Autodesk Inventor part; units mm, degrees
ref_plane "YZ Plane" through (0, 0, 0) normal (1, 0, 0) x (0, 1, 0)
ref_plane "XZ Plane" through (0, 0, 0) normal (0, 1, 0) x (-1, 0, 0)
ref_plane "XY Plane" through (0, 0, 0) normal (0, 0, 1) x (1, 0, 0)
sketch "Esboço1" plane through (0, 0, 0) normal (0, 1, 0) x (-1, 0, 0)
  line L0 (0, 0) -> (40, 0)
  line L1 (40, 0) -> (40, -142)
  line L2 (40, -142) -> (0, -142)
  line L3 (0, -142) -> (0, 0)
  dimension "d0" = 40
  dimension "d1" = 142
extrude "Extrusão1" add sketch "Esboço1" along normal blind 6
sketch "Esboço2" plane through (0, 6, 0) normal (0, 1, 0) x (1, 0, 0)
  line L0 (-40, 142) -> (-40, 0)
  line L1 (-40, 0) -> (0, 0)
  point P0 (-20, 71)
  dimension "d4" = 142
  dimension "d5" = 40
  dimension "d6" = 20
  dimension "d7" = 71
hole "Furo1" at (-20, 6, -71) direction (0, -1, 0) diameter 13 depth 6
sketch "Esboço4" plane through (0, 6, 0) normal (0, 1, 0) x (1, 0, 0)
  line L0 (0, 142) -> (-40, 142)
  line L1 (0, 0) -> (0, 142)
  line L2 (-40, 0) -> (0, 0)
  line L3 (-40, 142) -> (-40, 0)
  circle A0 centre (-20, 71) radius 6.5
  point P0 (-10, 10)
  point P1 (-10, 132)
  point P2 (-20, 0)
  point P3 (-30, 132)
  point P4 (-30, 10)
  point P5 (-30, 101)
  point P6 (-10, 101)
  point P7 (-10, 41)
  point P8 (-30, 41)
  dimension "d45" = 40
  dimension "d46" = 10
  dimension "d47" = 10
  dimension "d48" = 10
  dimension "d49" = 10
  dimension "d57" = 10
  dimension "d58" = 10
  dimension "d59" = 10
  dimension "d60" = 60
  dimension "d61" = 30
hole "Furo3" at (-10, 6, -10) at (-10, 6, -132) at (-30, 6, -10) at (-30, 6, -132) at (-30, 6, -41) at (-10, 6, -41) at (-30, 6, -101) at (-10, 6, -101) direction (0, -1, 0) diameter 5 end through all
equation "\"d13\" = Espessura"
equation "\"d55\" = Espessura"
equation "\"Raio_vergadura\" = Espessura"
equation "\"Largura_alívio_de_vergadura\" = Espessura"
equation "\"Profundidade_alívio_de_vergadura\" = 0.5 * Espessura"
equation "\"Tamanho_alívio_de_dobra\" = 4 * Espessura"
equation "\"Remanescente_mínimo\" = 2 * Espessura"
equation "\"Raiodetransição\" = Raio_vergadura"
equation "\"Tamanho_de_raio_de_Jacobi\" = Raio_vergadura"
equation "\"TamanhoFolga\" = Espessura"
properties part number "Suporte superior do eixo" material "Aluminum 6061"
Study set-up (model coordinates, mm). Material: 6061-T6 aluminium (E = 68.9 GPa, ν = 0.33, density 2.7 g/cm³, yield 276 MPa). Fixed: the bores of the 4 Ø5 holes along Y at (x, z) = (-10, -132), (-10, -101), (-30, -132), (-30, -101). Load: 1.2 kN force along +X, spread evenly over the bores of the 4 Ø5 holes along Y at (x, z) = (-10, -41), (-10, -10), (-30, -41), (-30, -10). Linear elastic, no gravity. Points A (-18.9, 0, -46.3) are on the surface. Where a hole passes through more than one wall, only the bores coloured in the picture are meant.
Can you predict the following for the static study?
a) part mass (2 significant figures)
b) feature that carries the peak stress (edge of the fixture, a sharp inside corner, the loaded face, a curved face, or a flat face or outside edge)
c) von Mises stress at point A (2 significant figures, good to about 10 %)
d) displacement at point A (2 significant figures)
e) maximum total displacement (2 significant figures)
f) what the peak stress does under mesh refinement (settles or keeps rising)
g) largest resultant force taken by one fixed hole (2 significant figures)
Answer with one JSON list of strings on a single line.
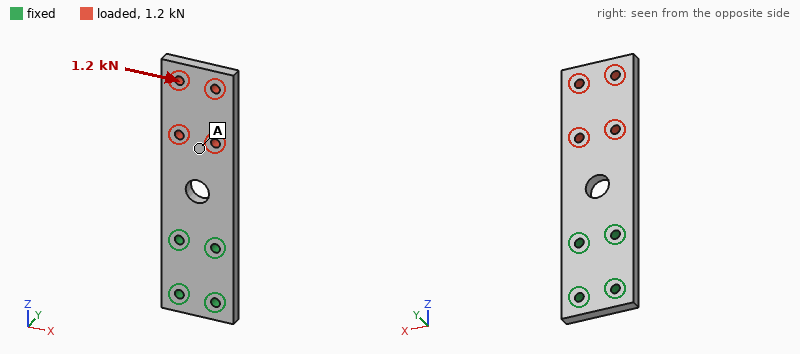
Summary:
["87 g", "edge of the fixture", "13 MPa", "0.074 mm", "0.17 mm", "keeps rising", "3.2 kN"]
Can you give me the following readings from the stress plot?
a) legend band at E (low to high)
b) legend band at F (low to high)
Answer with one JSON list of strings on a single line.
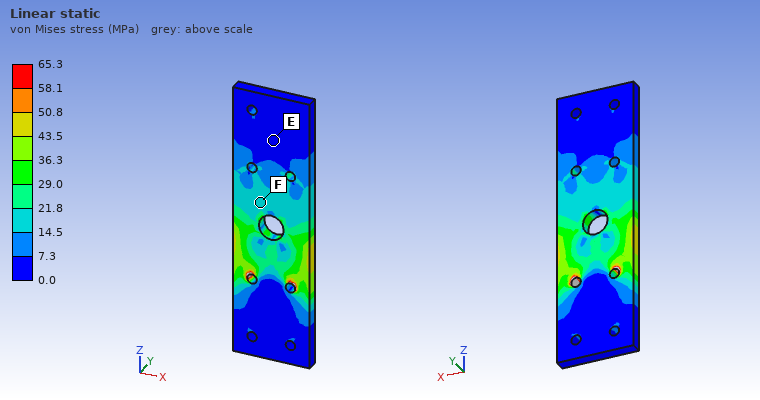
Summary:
["0.0 to 7.3 MPa", "14.5 to 21.8 MPa"]
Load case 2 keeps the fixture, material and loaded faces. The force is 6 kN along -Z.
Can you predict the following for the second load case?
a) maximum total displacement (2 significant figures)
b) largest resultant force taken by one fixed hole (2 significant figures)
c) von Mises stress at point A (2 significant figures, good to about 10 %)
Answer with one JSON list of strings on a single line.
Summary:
["35 µm", "2.7 kN", "19 MPa"]
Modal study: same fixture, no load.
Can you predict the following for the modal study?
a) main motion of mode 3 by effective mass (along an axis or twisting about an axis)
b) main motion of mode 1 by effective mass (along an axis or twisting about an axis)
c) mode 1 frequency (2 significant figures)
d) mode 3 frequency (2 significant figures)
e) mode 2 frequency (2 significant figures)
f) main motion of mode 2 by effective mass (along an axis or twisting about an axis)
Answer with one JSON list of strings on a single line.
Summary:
["along X", "along Y", "470 Hz", "2700 Hz", "2300 Hz", "twisting about Z"]
